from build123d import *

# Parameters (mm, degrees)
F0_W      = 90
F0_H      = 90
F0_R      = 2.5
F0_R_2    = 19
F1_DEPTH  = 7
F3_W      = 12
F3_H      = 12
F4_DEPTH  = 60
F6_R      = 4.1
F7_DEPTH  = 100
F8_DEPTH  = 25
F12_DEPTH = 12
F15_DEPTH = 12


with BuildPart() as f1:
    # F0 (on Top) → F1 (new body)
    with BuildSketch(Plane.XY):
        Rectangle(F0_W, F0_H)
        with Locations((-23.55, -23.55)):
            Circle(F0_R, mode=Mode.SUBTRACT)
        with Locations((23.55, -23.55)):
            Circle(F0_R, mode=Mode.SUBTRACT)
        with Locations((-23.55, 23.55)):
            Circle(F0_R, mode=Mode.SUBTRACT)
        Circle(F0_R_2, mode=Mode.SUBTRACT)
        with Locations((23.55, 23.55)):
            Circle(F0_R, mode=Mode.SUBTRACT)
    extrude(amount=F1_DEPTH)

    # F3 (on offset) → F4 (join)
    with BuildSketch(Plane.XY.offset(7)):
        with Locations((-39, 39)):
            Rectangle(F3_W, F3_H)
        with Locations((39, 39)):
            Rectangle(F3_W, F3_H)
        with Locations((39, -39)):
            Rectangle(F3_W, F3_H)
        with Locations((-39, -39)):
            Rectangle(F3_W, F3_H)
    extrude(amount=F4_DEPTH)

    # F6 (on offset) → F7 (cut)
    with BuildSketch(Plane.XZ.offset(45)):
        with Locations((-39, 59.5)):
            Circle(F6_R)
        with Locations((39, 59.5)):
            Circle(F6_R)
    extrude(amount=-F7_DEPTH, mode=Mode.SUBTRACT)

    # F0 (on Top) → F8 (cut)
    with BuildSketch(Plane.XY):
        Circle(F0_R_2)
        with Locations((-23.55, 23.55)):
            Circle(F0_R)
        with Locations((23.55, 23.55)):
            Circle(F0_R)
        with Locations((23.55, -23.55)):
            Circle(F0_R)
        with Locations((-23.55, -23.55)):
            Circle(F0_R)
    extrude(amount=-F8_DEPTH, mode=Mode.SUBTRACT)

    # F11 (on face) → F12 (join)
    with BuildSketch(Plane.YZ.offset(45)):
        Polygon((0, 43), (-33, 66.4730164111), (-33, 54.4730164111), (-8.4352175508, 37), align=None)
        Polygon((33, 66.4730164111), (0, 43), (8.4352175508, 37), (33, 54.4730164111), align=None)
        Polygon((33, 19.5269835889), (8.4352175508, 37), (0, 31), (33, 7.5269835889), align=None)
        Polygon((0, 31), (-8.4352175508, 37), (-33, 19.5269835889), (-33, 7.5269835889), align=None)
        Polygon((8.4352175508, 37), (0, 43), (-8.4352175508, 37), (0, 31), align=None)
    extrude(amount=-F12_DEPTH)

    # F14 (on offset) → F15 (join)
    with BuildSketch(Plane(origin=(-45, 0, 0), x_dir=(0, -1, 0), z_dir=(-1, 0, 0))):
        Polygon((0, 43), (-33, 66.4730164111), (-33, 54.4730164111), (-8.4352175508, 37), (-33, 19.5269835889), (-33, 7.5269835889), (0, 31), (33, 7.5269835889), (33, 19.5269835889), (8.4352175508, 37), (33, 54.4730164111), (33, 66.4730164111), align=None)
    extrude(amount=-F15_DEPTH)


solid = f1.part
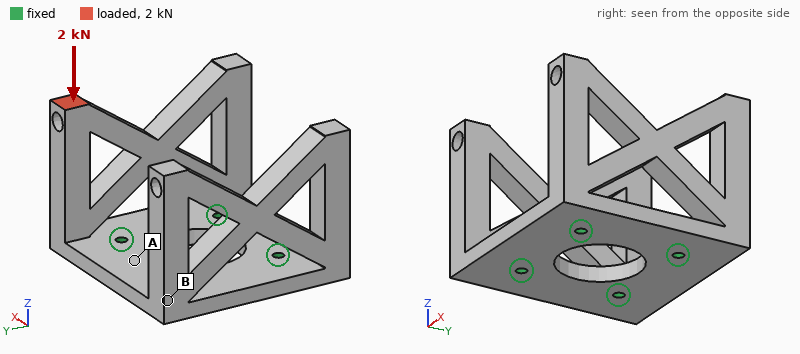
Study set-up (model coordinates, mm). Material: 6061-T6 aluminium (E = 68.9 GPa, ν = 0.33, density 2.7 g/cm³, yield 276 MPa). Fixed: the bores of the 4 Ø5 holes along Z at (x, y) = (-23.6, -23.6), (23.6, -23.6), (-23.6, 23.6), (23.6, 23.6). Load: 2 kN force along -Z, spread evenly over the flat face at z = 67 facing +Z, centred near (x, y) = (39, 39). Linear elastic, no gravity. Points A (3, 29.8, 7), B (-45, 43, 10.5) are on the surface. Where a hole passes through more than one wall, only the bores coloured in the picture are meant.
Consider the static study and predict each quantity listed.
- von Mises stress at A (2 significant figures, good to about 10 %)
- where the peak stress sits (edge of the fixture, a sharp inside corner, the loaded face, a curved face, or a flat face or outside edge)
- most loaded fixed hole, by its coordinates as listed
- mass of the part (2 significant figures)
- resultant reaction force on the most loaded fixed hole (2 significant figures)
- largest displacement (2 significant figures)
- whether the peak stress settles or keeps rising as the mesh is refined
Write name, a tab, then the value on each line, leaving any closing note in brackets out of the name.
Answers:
von Mises stress at A	12 MPa
where the peak stress sits	edge of the fixture
most loaded fixed hole, by its coordinates as listed	(23.6, 23.6)
mass of the part	310 g
resultant reaction force on the most loaded fixed hole	2.4 kN
largest displacement	0.25 mm
whether the peak stress settles or keeps rising as the mesh is refined	keeps rising
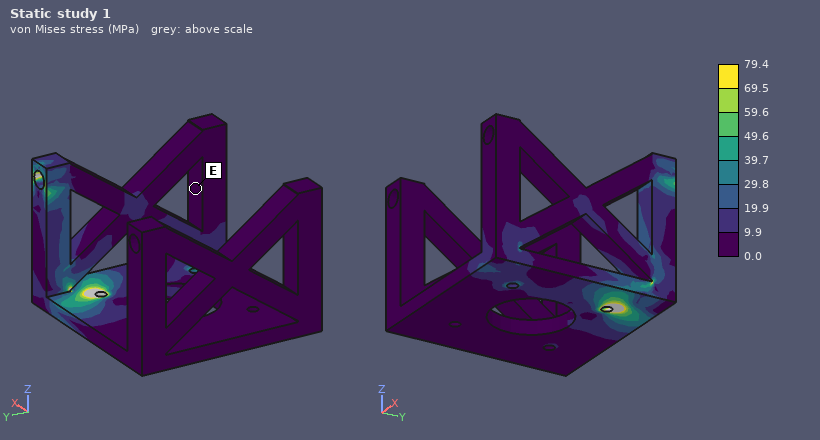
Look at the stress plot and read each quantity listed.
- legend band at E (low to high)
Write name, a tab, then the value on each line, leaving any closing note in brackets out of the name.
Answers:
legend band at E	0.0 to 9.9 MPa
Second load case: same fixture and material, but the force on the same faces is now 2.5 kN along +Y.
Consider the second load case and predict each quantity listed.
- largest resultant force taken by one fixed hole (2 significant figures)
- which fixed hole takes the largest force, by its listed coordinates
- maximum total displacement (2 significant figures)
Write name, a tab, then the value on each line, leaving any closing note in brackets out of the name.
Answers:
largest resultant force taken by one fixed hole	3.2 kN
which fixed hole takes the largest force, by its listed coordinates	(23.6, -23.6)
maximum total displacement	0.28 mm
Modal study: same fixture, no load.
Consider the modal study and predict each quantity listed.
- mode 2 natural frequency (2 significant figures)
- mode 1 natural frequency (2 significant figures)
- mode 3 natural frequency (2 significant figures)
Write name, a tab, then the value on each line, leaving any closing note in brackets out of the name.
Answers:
mode 2 natural frequency	1000 Hz
mode 1 natural frequency	1000 Hz
mode 3 natural frequency	2200 Hz
